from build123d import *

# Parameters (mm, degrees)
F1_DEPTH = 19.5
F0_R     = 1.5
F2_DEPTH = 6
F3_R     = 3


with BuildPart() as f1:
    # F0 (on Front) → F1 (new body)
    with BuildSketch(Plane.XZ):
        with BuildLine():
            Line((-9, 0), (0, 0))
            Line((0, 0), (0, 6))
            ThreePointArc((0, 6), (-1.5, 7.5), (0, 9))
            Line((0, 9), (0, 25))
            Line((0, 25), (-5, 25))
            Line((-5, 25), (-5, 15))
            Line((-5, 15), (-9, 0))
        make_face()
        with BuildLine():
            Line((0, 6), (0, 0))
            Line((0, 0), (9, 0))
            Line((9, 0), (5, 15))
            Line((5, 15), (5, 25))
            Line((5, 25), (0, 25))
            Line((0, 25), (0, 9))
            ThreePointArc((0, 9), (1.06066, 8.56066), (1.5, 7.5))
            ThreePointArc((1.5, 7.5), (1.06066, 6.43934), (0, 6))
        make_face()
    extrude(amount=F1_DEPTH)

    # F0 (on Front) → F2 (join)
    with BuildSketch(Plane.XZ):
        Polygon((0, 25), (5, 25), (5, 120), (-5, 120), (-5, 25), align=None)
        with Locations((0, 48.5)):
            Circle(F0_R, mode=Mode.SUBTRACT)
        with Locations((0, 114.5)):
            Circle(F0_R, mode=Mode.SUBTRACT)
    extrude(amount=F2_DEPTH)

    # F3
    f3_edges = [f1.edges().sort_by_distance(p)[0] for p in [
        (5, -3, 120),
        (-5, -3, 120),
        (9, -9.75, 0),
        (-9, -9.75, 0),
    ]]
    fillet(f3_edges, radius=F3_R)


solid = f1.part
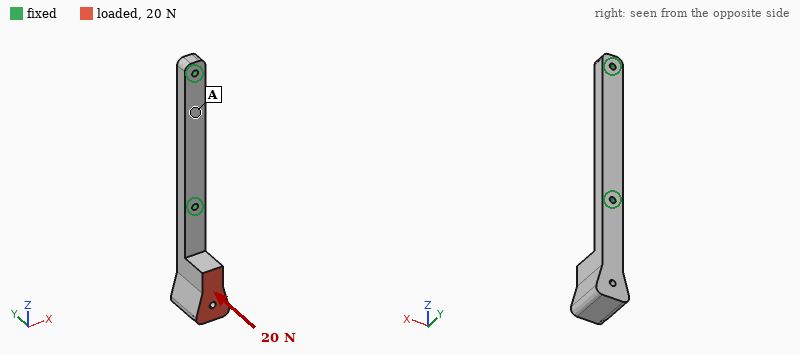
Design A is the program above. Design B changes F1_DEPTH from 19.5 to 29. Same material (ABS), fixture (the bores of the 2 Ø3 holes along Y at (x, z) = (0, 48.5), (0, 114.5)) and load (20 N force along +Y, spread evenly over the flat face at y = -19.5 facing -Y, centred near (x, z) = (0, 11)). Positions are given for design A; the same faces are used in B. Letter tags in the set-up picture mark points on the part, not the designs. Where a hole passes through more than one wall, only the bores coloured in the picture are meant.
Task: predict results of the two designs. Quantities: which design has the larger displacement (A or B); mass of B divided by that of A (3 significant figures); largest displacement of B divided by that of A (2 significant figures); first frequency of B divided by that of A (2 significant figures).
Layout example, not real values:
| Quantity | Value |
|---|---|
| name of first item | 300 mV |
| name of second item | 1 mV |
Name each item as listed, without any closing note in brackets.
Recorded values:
| Quantity | Value |
|---|---|
| which design has the larger displacement | B |
| mass of B divided by that of A | 1.25 |
| largest displacement of B divided by that of A | 1.1 |
| first frequency of B divided by that of A | 0.76 |
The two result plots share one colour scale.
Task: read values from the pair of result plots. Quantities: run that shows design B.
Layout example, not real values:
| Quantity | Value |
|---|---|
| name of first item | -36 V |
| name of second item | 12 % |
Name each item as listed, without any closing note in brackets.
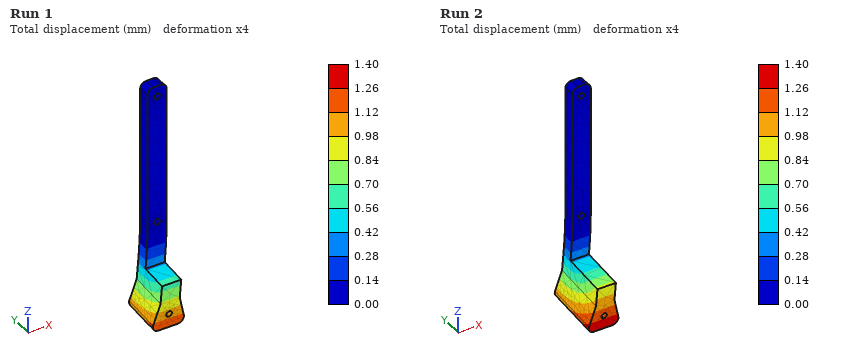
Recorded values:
| Quantity | Value |
|---|---|
| run that shows design B | Run 2 |
